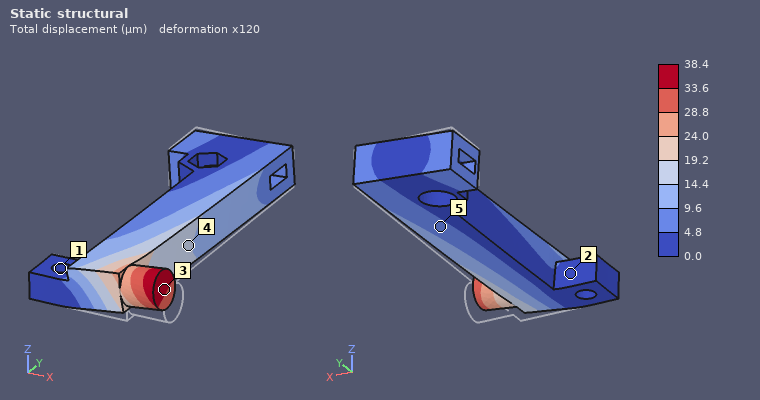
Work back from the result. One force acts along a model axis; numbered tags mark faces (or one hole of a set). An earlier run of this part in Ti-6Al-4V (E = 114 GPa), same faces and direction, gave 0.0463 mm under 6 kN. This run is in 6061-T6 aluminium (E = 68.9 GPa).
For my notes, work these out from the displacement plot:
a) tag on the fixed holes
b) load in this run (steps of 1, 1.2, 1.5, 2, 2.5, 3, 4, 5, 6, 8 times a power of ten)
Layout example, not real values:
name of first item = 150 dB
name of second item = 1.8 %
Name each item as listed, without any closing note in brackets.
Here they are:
tag on the fixed holes = 1
load in this run = 3 kN
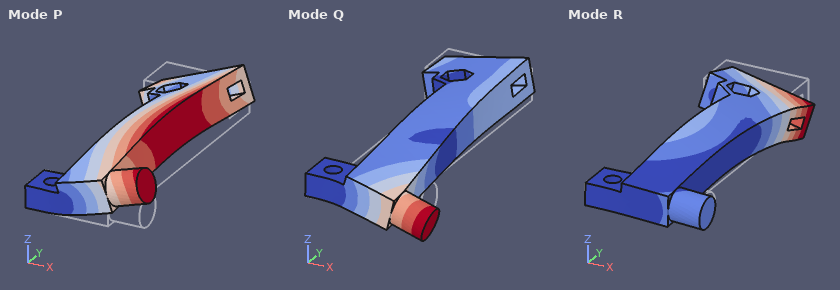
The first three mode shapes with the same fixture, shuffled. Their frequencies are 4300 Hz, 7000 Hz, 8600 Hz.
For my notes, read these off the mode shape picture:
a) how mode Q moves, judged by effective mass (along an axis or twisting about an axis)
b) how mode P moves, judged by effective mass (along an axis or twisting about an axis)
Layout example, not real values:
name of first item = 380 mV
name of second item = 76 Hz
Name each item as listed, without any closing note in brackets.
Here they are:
how mode Q moves, judged by effective mass = twisting about X
how mode P moves, judged by effective mass = along Z
